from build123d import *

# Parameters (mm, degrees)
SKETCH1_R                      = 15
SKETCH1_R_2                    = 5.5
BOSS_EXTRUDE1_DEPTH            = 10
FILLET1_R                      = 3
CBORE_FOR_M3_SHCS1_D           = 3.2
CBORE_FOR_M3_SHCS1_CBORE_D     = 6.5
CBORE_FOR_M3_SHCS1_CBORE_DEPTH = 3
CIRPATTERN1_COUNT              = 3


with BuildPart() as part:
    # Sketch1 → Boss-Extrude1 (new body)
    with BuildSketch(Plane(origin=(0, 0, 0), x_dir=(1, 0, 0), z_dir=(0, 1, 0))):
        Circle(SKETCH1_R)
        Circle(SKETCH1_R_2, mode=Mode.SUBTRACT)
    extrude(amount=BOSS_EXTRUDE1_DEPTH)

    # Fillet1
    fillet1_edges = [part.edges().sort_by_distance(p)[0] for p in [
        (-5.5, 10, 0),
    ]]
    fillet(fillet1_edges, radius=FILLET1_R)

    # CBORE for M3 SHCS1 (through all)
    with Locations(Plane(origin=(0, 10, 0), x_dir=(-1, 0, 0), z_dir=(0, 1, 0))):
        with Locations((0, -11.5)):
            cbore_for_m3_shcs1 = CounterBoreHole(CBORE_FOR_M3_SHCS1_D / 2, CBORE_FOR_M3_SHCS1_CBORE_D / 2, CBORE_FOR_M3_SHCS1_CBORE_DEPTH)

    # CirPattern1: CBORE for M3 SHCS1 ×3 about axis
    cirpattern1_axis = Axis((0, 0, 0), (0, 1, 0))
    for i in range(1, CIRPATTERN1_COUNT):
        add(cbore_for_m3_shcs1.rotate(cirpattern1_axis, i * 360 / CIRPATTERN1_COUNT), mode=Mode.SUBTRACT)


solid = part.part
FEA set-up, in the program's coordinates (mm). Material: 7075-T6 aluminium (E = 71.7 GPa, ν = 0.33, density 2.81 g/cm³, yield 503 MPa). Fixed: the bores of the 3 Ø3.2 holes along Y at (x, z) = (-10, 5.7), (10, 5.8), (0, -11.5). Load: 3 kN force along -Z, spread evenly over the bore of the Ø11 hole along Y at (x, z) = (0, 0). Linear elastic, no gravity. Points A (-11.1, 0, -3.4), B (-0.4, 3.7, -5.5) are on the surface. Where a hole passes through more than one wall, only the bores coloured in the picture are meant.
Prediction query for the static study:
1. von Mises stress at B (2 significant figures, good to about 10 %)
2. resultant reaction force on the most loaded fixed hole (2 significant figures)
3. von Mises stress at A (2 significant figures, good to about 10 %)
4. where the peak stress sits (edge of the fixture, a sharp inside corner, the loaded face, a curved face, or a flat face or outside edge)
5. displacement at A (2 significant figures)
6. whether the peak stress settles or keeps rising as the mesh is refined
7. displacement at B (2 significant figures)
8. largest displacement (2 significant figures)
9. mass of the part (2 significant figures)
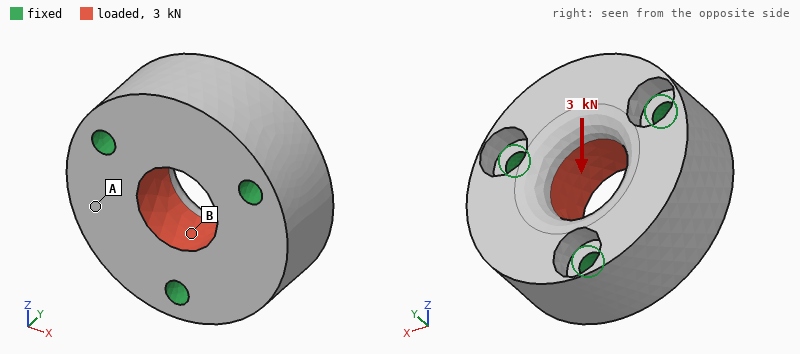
20 MPa
1.1 kN
5.9 MPa
edge of the fixture
1.1 µm
keeps rising
1.1 µm
3.2 µm
16 g
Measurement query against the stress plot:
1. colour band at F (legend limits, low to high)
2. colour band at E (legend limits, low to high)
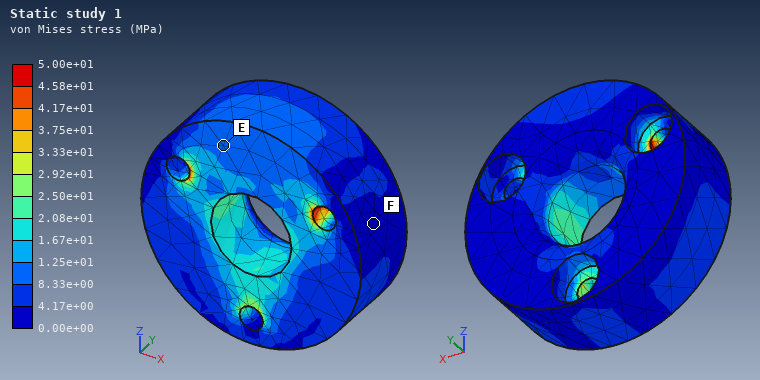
0.00e+00 to 4.17e+00 MPa
8.33e+00 to 1.25e+01 MPa
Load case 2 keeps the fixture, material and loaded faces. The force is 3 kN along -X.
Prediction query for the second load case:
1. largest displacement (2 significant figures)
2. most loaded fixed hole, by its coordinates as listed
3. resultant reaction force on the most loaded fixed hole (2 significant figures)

2.9 µm
(0, -11.5)
1.1 kN
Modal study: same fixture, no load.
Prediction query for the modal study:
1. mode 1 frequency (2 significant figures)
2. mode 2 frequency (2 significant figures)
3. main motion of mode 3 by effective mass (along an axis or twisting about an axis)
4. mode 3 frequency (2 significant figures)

37 kHz
37 kHz
along Y
44 kHz
